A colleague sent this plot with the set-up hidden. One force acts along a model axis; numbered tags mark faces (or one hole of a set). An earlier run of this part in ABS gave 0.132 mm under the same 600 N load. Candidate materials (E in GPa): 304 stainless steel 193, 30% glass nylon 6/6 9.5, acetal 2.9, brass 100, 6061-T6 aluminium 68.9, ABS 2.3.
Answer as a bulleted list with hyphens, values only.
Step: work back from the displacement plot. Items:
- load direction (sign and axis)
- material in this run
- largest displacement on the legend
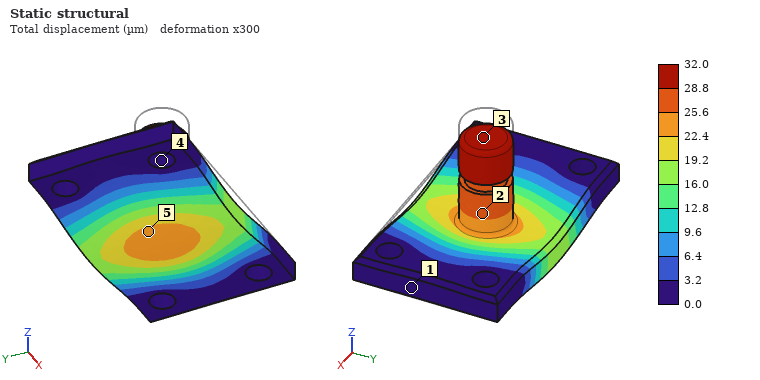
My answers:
- -Z
- 30% glass nylon 6/6
- 32.0 µm
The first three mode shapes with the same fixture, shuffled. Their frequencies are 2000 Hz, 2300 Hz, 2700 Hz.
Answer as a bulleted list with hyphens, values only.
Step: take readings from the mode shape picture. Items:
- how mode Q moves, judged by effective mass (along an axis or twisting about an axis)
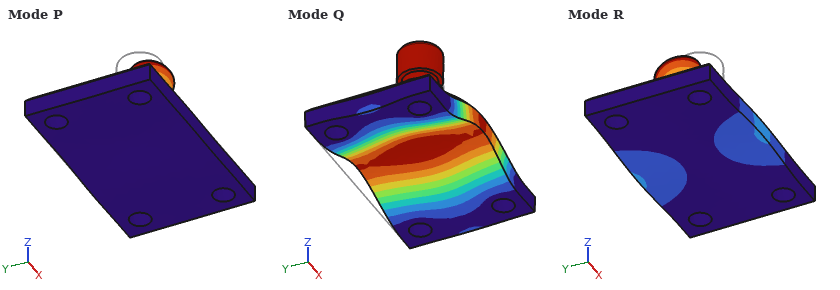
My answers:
- along Z
